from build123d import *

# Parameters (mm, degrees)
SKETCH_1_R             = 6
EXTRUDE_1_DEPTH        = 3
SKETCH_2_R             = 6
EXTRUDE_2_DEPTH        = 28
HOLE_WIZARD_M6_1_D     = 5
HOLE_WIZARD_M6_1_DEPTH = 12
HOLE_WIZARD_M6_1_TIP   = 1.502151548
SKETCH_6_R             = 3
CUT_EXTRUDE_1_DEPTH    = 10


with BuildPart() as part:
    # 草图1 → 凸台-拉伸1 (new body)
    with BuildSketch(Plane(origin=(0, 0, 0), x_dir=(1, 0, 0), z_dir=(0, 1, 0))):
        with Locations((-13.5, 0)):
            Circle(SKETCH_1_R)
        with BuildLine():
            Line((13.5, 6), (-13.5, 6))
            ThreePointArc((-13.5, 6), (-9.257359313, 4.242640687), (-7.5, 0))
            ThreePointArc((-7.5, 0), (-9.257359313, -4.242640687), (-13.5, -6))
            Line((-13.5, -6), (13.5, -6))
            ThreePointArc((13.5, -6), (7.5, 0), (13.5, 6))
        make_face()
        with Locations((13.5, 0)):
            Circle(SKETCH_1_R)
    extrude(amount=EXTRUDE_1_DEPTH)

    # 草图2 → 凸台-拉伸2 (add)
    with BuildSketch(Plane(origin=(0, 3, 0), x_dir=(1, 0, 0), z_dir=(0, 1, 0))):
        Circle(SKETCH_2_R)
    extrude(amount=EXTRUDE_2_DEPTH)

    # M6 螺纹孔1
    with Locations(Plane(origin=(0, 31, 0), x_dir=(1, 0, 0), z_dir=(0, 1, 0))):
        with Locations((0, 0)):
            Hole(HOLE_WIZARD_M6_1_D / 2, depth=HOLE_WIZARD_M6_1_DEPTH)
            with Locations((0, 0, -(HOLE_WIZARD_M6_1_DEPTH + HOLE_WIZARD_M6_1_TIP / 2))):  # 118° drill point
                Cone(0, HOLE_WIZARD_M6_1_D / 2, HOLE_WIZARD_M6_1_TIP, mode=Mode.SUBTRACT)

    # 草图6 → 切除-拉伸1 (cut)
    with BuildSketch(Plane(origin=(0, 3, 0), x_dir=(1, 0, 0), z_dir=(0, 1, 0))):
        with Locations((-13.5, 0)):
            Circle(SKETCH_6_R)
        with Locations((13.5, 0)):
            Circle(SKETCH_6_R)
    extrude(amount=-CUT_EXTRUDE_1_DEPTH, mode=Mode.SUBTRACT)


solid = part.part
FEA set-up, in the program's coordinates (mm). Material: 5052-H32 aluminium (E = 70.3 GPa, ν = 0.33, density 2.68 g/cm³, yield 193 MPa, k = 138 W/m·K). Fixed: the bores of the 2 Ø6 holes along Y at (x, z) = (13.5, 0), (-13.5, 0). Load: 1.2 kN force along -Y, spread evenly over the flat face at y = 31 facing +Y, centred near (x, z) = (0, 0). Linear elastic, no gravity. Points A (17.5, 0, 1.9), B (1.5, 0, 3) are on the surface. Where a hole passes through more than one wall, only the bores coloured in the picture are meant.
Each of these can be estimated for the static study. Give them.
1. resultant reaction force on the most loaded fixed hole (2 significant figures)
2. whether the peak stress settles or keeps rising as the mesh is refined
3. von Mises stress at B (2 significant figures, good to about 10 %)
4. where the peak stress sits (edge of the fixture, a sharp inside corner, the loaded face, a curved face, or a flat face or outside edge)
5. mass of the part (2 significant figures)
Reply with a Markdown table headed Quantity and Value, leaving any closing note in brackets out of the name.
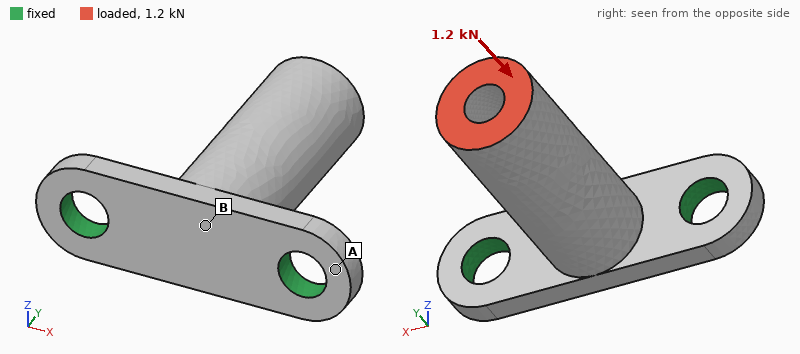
| Quantity | Value |
|---|---|
| resultant reaction force on the most loaded fixed hole | 650 N |
| whether the peak stress settles or keeps rising as the mesh is refined | keeps rising |
| von Mises stress at B | 31 MPa |
| where the peak stress sits | edge of the fixture |
| mass of the part | 11 g |
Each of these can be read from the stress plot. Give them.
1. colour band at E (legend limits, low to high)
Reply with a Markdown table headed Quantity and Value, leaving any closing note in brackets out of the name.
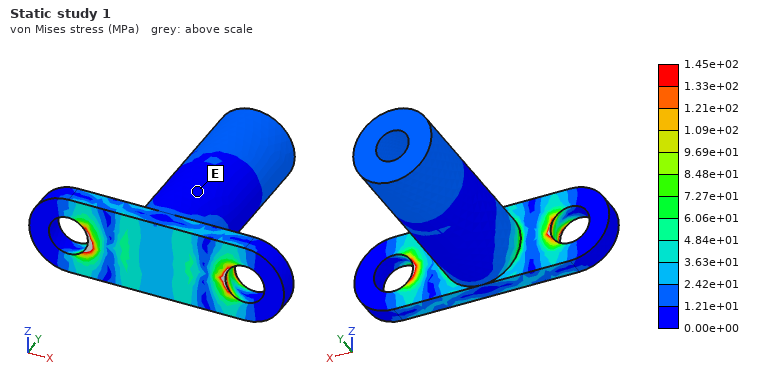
| Quantity | Value |
|---|---|
| colour band at E | 0.00e+00 to 1.21e+01 MPa |
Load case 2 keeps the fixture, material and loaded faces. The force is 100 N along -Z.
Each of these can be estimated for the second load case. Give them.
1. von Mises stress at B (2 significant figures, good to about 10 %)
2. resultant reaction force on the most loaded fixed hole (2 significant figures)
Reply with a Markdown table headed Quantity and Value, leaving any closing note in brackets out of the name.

| Quantity | Value |
|---|---|
| von Mises stress at B | 19 MPa |
| resultant reaction force on the most loaded fixed hole | 50 N |
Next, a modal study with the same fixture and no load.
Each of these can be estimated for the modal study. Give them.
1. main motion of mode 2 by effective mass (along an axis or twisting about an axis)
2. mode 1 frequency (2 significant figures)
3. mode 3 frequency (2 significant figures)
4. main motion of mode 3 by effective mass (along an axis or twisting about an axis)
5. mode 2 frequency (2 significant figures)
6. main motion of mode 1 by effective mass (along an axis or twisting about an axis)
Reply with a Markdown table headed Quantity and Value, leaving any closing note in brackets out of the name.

| Quantity | Value |
|---|---|
| main motion of mode 2 by effective mass | along X |
| mode 1 frequency | 3100 Hz |
| mode 3 frequency | 14 kHz |
| main motion of mode 3 by effective mass | along Y |
| mode 2 frequency | 6300 Hz |
| main motion of mode 1 by effective mass | along Z |
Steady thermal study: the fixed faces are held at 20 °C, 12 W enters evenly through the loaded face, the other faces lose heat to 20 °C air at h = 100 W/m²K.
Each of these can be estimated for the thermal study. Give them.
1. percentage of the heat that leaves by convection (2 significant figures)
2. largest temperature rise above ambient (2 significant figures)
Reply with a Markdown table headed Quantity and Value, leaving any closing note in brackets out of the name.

| Quantity | Value |
|---|---|
| percentage of the heat that leaves by convection | 22 % |
| largest temperature rise above ambient | 29 K |
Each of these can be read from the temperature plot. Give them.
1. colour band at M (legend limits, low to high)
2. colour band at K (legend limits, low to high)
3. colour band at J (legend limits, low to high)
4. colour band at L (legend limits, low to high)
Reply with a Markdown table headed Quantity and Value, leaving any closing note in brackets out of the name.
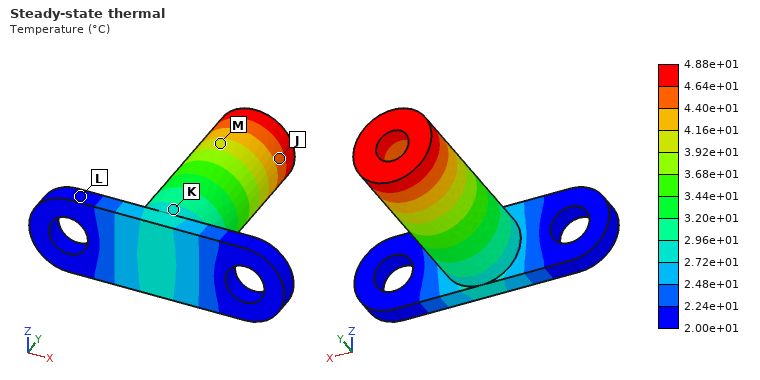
| Quantity | Value |
|---|---|
| colour band at M | 3.92e+01 to 4.16e+01 °C |
| colour band at K | 2.72e+01 to 2.96e+01 °C |
| colour band at J | 4.40e+01 to 4.64e+01 °C |
| colour band at L | 2.00e+01 to 2.24e+01 °C |
